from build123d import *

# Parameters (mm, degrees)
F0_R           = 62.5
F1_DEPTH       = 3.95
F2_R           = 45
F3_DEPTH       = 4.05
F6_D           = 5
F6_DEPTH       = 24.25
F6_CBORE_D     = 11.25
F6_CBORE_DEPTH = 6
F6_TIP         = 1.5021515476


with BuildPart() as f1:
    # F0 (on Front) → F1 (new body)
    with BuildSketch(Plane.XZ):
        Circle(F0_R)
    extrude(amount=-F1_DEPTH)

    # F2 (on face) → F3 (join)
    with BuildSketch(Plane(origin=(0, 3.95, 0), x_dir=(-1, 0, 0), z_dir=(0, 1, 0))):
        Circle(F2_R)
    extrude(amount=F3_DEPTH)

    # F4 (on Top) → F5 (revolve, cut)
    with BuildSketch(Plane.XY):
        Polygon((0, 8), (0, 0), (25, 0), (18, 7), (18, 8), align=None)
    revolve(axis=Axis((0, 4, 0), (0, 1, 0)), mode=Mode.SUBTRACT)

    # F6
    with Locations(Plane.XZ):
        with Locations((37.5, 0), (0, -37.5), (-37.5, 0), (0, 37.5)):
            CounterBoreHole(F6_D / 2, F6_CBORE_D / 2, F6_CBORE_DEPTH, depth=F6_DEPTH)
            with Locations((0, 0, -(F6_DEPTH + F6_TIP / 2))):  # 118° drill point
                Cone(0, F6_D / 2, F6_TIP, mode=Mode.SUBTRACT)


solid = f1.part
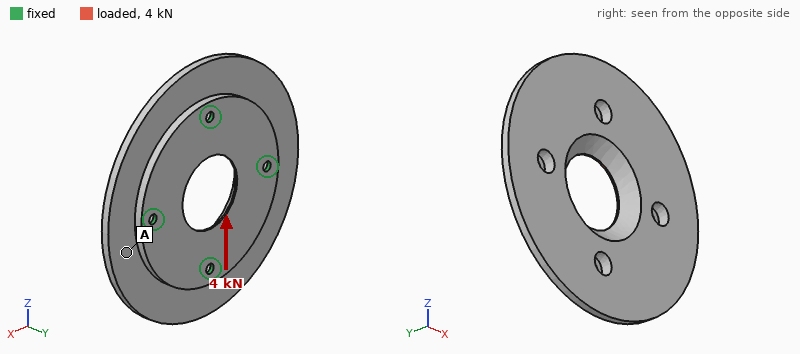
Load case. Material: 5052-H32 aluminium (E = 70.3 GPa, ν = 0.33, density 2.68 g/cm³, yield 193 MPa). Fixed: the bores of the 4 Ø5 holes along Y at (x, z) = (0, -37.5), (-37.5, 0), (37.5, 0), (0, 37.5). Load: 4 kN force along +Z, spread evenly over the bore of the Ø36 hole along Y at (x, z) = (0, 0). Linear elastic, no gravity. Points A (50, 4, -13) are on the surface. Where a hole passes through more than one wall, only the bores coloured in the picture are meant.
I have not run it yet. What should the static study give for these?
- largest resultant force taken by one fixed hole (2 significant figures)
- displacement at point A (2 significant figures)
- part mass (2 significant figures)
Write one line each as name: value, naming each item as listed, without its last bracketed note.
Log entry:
largest resultant force taken by one fixed hole: 1.0 kN
displacement at point A: 2.7 µm
part mass: 160 g
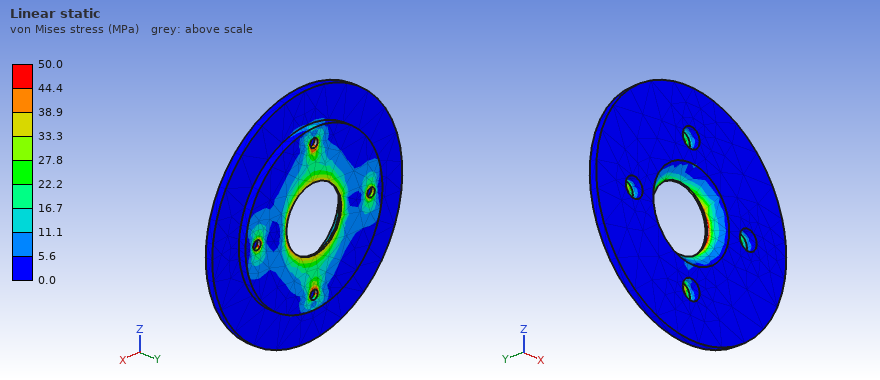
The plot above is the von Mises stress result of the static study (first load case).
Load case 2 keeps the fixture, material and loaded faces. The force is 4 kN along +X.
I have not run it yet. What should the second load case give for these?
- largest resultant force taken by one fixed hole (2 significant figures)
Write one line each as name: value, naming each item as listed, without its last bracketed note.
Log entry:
largest resultant force taken by one fixed hole: 1.0 kN
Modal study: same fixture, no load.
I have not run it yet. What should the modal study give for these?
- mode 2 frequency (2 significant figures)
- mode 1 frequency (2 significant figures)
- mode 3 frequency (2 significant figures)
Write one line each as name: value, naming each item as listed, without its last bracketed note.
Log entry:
mode 2 frequency: 3800 Hz
mode 1 frequency: 3100 Hz
mode 3 frequency: 3800 Hz
